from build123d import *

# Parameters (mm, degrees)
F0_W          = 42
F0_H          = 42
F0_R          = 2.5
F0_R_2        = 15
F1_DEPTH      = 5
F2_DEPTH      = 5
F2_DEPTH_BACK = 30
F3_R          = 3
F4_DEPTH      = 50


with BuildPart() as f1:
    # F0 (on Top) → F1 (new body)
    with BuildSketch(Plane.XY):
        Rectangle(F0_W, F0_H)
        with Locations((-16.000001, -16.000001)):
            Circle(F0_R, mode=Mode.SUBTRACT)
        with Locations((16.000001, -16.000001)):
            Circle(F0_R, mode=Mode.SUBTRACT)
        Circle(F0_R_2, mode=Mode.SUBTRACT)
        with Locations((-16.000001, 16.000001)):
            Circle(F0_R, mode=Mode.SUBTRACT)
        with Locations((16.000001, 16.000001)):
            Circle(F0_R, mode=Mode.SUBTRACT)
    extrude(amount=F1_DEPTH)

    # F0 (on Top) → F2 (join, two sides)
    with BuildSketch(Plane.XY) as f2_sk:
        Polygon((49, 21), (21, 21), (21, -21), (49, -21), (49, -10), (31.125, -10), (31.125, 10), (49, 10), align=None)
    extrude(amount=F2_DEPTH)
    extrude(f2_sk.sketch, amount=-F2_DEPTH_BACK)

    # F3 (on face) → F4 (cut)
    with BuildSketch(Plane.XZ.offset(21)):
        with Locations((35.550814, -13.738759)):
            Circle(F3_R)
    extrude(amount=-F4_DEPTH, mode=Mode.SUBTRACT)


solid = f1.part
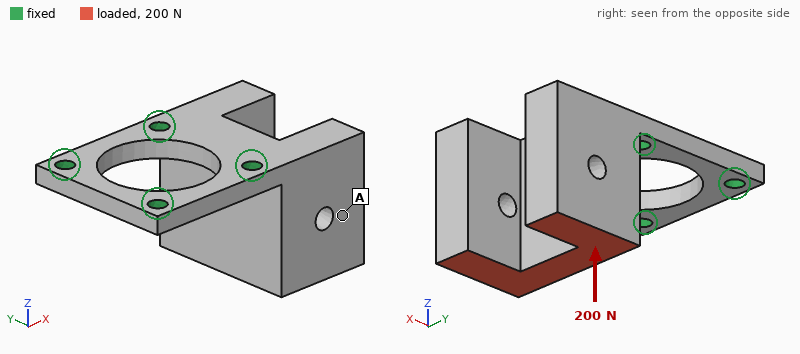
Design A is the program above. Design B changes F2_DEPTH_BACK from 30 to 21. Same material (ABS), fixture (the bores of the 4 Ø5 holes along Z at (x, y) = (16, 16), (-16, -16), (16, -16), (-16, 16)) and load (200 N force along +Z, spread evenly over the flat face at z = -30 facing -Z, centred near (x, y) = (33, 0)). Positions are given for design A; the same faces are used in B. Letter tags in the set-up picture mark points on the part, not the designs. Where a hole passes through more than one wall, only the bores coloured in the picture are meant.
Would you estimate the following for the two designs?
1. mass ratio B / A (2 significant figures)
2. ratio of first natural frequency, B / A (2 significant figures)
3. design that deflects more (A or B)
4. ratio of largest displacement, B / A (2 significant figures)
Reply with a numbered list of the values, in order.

1. 0.78
2. 1.4
3. A
4. 0.87
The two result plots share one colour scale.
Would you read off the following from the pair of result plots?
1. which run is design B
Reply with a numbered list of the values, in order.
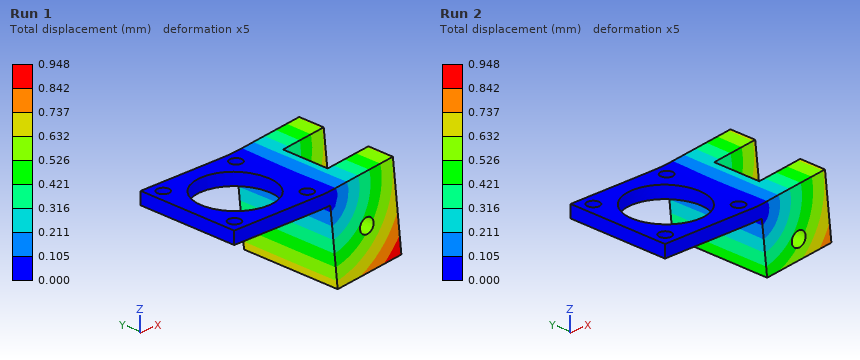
1. Run 2
